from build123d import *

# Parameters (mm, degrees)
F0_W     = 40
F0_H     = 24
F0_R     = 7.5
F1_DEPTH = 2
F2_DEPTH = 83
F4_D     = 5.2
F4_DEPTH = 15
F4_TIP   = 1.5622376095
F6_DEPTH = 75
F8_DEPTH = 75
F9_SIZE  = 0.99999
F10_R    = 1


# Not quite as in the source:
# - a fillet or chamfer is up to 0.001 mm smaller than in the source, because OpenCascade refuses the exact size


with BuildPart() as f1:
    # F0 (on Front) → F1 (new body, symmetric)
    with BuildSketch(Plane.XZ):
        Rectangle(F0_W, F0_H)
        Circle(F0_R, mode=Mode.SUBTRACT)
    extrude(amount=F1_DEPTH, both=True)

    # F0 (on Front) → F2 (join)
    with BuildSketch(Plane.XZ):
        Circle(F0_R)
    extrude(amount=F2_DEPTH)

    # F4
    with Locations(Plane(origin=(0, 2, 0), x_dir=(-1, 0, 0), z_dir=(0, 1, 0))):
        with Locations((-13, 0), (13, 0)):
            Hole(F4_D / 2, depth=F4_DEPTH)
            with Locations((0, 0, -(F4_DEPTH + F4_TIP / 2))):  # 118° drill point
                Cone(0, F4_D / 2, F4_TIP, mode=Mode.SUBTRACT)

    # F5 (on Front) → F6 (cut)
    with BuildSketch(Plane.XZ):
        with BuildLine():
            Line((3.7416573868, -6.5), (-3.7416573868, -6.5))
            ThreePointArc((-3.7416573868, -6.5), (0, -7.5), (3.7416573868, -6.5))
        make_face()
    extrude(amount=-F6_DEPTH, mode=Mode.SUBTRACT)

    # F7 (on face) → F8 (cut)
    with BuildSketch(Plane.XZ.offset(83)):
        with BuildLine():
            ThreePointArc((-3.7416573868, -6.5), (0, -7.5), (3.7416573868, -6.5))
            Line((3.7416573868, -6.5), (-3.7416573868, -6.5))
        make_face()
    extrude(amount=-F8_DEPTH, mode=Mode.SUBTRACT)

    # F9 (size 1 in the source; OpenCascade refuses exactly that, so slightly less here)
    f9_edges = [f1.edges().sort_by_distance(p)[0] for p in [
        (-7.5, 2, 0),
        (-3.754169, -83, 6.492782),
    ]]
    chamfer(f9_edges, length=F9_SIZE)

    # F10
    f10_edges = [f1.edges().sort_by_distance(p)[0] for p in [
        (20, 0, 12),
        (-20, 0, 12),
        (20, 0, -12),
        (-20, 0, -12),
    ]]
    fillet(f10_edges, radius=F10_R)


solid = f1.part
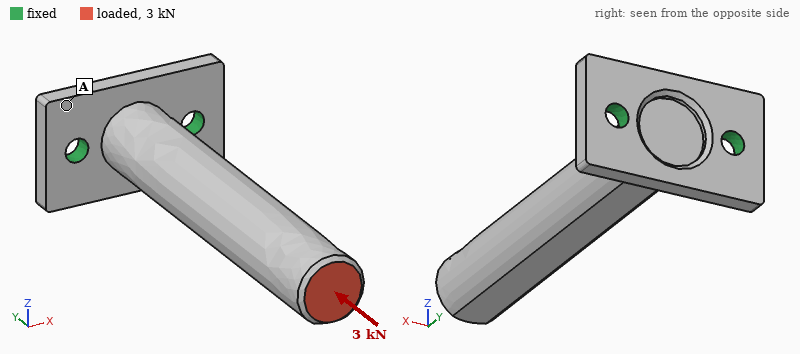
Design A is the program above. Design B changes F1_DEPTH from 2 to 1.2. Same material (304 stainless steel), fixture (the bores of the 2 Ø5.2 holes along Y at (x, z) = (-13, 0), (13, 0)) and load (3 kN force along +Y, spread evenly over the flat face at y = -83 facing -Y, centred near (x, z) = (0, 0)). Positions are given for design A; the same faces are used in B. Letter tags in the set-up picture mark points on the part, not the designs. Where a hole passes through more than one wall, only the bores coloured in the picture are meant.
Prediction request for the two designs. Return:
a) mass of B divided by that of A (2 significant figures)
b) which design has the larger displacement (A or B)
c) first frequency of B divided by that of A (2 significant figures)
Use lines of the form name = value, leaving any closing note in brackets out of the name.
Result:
mass of B divided by that of A = 0.93
which design has the larger displacement = B
first frequency of B divided by that of A = 0.61
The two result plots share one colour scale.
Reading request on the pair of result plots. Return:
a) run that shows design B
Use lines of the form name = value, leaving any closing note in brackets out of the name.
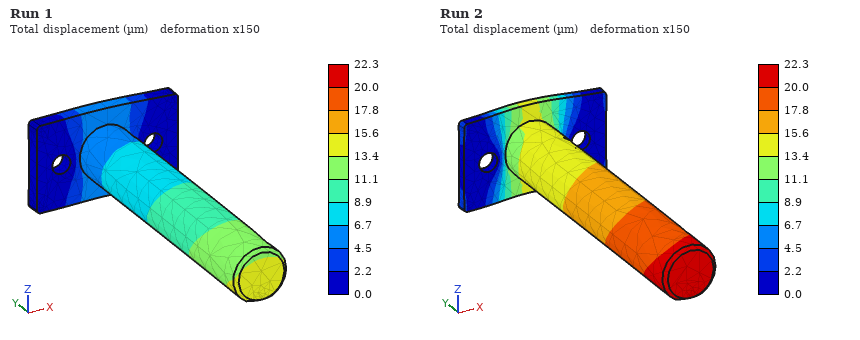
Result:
run that shows design B = Run 2
